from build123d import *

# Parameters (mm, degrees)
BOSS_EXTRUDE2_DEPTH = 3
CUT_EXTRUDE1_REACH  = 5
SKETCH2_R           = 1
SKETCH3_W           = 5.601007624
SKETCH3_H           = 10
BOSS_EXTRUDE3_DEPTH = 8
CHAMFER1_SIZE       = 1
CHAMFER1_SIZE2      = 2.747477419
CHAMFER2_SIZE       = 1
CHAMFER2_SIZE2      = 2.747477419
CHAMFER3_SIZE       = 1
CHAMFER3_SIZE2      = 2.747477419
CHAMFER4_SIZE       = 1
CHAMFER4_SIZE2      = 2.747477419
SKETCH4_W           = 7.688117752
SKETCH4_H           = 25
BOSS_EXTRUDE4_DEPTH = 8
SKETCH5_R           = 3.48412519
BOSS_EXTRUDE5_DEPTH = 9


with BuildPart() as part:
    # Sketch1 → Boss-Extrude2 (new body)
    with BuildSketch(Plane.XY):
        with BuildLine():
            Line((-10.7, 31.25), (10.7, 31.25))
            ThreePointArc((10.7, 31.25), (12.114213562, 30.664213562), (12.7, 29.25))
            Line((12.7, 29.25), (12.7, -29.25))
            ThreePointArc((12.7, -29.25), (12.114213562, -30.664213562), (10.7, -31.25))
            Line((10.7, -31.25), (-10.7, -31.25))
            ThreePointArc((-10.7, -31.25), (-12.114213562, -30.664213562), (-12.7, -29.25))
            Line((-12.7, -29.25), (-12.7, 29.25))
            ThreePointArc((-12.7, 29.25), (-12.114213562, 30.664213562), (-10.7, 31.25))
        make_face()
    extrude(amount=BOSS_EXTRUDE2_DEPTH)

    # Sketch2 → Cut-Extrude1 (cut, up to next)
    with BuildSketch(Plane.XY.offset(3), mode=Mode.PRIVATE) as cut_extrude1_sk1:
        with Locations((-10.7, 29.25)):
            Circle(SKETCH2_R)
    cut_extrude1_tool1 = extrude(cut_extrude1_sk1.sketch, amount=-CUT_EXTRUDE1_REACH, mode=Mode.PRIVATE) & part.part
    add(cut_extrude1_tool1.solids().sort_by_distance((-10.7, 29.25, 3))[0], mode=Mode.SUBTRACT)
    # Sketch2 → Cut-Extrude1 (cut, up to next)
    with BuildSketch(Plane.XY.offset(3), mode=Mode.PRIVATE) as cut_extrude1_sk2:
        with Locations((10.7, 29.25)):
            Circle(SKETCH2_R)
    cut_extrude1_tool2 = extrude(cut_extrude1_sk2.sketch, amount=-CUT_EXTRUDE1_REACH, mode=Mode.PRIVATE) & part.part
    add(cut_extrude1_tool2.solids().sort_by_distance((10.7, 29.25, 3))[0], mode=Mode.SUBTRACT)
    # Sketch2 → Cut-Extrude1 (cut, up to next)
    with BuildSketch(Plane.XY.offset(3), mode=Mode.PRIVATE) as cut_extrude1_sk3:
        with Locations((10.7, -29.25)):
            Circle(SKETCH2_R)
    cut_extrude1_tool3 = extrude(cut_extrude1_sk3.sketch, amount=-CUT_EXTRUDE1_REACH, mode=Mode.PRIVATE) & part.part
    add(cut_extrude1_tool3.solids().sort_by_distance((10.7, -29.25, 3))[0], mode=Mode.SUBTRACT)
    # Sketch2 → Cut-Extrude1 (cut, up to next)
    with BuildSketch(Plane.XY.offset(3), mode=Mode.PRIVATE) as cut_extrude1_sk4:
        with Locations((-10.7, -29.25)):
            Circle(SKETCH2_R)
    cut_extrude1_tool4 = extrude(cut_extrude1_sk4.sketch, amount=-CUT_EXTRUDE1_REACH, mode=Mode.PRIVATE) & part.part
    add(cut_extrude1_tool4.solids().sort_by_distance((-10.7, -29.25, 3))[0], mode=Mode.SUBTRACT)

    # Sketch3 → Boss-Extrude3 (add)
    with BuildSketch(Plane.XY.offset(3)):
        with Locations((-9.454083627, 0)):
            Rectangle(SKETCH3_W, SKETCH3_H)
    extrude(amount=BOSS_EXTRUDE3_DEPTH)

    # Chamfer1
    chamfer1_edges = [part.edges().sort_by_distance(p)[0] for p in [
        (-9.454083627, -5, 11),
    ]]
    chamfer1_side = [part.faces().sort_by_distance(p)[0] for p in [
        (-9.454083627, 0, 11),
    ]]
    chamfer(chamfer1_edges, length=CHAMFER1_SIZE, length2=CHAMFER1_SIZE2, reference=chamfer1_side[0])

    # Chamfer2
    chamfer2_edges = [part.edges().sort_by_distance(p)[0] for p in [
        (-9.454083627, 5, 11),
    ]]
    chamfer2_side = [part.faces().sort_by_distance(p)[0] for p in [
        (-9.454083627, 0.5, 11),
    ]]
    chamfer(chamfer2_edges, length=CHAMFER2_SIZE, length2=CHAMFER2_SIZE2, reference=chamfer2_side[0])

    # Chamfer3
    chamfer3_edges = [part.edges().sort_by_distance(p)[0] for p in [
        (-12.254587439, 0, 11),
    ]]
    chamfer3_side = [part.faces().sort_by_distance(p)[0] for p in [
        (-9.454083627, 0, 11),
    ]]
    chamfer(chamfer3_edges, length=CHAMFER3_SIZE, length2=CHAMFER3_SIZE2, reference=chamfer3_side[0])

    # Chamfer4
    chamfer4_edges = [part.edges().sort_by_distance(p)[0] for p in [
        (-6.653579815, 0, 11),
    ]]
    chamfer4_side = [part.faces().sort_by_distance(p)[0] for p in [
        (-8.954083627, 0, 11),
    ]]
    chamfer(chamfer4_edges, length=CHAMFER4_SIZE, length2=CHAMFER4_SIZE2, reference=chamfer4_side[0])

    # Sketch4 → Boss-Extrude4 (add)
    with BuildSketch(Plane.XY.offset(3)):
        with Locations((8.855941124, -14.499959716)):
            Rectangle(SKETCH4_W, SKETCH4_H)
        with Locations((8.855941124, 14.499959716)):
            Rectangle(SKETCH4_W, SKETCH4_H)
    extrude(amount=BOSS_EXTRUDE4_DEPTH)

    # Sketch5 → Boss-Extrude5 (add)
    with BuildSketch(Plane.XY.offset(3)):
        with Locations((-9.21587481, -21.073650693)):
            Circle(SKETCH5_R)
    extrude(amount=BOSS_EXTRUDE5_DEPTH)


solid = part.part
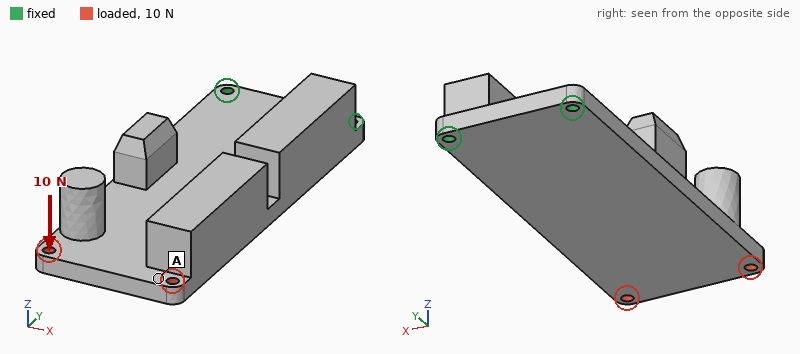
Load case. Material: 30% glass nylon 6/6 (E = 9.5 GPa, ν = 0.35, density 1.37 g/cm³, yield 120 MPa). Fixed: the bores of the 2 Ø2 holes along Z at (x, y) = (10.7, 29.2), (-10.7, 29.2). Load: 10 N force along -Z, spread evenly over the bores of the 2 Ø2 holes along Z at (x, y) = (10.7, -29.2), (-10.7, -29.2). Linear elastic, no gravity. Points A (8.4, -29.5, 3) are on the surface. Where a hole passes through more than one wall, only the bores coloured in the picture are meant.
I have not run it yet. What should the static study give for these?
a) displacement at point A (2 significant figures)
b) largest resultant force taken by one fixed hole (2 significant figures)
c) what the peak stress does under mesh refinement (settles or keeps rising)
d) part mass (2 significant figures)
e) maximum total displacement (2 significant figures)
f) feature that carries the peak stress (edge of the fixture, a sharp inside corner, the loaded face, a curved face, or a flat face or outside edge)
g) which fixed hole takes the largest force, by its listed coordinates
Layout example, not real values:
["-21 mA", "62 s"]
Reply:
["0.71 mm", "7.4 N", "keeps rising", "12 g", "0.76 mm", "edge of the fixture", "(-10.7, 29.2)"]
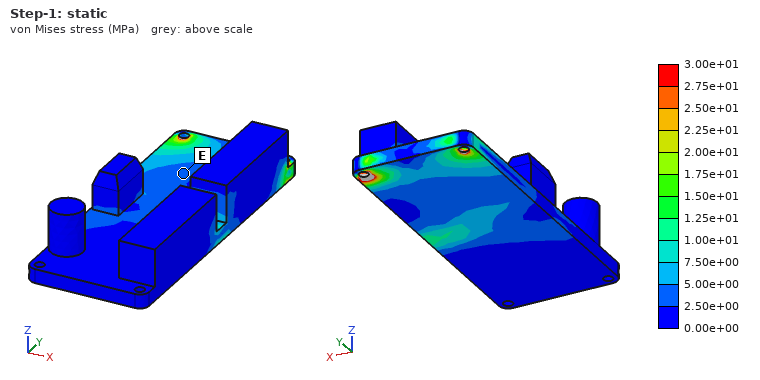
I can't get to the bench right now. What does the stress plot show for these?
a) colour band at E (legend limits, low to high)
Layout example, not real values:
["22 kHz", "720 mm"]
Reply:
["2.50e+00 to 5.00e+00 MPa"]
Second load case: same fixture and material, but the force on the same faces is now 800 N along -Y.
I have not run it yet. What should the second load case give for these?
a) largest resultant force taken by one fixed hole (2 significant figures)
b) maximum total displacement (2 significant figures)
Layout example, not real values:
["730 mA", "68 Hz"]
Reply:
["420 N", "0.25 mm"]
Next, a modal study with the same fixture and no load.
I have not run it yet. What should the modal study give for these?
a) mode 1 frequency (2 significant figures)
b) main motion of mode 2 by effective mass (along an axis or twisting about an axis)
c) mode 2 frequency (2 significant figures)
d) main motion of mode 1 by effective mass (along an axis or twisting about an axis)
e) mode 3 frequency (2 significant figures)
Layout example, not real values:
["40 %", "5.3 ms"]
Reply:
["320 Hz", "along X", "1500 Hz", "along Z", "2000 Hz"]
